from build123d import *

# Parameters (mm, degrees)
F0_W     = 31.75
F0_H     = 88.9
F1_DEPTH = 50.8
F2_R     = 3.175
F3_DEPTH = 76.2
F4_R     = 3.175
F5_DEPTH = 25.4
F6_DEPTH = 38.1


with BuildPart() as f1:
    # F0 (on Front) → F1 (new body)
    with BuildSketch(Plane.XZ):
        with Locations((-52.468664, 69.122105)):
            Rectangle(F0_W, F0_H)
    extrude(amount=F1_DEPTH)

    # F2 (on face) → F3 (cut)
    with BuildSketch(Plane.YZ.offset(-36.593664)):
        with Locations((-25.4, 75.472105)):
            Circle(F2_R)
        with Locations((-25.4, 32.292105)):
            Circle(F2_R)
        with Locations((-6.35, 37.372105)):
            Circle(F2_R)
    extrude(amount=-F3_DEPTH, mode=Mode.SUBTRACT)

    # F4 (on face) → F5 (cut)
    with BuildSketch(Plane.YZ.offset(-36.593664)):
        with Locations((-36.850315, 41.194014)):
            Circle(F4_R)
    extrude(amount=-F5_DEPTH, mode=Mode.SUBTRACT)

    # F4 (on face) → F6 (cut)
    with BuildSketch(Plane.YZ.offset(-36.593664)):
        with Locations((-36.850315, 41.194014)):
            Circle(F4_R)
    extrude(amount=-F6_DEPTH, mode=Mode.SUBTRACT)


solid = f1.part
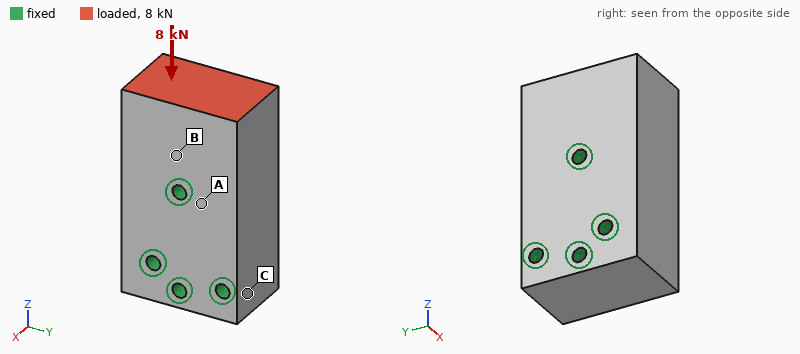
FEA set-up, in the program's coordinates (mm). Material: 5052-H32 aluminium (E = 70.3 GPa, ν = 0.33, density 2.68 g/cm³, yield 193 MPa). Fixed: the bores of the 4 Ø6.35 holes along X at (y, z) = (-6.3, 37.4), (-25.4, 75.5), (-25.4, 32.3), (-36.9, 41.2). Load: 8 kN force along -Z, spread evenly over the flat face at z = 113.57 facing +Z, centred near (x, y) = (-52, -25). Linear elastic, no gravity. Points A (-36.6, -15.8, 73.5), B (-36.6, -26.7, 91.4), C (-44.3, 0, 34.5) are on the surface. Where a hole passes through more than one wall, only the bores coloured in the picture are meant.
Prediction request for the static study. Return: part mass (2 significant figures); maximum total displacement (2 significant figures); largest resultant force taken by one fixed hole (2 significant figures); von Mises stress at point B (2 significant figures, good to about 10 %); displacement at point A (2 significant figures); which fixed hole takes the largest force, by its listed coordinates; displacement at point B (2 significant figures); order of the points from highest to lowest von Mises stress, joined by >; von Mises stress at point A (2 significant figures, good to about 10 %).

370 g
3.7 µm
5.4 kN
6.7 MPa
0.83 µm
(-25.4, 75.5)
1.7 µm
B > A > C
3.9 MPa
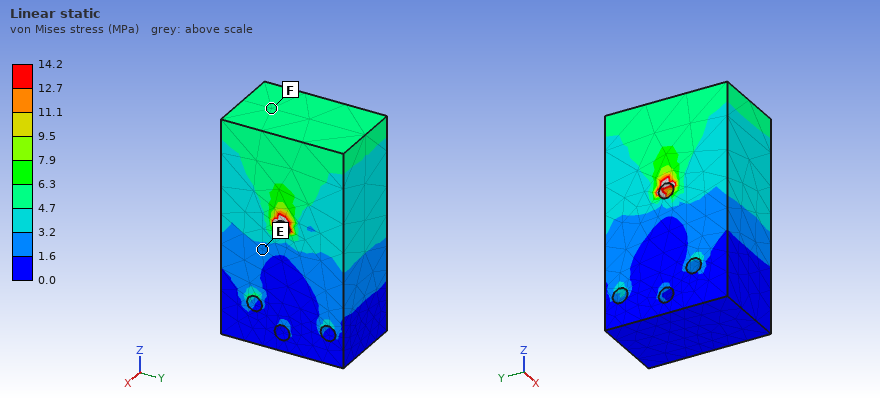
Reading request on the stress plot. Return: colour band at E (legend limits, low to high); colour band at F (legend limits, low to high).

1.6 to 3.2 MPa
4.7 to 6.3 MPa
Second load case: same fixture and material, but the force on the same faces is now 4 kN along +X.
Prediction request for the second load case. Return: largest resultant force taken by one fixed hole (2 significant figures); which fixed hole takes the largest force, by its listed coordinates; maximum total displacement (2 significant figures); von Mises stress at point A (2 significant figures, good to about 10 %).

5.1 kN
(-25.4, 75.5)
18 µm
12 MPa
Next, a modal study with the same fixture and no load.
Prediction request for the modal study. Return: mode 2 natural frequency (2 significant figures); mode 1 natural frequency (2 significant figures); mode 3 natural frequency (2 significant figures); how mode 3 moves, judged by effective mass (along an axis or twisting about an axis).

11 kHz
10 kHz
14 kHz
twisting about Z
